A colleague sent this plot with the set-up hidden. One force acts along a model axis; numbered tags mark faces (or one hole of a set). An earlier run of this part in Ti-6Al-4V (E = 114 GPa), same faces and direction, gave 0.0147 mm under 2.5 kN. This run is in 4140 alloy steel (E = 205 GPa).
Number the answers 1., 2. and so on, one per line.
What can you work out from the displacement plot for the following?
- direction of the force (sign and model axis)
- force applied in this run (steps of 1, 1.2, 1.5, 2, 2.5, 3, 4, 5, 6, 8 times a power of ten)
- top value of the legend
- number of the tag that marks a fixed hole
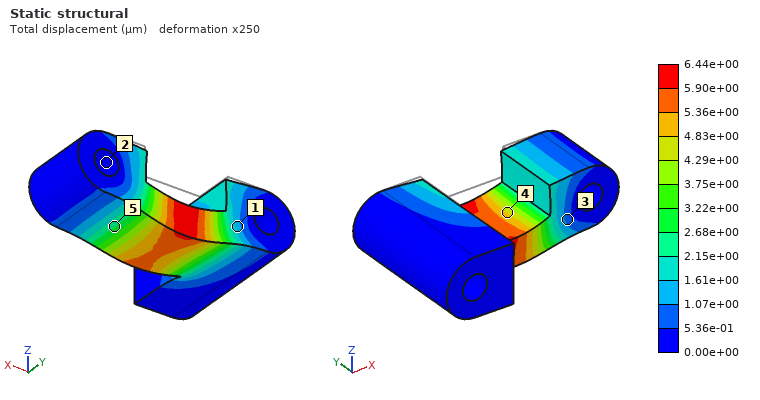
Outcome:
1. -Z
2. 2 kN
3. 6.44e+00 µm
4. 2
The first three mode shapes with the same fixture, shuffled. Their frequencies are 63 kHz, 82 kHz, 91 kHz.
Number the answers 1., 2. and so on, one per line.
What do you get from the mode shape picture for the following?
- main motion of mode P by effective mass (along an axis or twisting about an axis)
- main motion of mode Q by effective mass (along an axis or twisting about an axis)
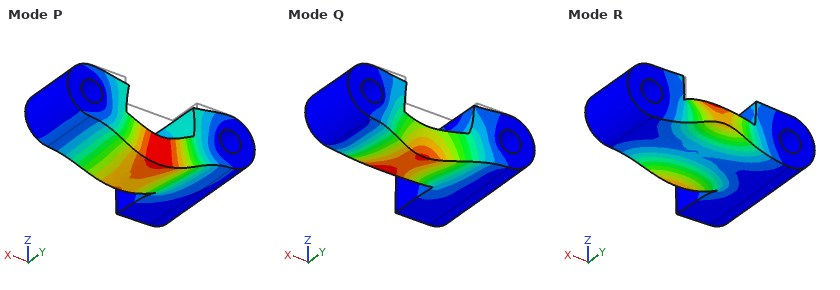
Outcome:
1. along Z
2. along Y
